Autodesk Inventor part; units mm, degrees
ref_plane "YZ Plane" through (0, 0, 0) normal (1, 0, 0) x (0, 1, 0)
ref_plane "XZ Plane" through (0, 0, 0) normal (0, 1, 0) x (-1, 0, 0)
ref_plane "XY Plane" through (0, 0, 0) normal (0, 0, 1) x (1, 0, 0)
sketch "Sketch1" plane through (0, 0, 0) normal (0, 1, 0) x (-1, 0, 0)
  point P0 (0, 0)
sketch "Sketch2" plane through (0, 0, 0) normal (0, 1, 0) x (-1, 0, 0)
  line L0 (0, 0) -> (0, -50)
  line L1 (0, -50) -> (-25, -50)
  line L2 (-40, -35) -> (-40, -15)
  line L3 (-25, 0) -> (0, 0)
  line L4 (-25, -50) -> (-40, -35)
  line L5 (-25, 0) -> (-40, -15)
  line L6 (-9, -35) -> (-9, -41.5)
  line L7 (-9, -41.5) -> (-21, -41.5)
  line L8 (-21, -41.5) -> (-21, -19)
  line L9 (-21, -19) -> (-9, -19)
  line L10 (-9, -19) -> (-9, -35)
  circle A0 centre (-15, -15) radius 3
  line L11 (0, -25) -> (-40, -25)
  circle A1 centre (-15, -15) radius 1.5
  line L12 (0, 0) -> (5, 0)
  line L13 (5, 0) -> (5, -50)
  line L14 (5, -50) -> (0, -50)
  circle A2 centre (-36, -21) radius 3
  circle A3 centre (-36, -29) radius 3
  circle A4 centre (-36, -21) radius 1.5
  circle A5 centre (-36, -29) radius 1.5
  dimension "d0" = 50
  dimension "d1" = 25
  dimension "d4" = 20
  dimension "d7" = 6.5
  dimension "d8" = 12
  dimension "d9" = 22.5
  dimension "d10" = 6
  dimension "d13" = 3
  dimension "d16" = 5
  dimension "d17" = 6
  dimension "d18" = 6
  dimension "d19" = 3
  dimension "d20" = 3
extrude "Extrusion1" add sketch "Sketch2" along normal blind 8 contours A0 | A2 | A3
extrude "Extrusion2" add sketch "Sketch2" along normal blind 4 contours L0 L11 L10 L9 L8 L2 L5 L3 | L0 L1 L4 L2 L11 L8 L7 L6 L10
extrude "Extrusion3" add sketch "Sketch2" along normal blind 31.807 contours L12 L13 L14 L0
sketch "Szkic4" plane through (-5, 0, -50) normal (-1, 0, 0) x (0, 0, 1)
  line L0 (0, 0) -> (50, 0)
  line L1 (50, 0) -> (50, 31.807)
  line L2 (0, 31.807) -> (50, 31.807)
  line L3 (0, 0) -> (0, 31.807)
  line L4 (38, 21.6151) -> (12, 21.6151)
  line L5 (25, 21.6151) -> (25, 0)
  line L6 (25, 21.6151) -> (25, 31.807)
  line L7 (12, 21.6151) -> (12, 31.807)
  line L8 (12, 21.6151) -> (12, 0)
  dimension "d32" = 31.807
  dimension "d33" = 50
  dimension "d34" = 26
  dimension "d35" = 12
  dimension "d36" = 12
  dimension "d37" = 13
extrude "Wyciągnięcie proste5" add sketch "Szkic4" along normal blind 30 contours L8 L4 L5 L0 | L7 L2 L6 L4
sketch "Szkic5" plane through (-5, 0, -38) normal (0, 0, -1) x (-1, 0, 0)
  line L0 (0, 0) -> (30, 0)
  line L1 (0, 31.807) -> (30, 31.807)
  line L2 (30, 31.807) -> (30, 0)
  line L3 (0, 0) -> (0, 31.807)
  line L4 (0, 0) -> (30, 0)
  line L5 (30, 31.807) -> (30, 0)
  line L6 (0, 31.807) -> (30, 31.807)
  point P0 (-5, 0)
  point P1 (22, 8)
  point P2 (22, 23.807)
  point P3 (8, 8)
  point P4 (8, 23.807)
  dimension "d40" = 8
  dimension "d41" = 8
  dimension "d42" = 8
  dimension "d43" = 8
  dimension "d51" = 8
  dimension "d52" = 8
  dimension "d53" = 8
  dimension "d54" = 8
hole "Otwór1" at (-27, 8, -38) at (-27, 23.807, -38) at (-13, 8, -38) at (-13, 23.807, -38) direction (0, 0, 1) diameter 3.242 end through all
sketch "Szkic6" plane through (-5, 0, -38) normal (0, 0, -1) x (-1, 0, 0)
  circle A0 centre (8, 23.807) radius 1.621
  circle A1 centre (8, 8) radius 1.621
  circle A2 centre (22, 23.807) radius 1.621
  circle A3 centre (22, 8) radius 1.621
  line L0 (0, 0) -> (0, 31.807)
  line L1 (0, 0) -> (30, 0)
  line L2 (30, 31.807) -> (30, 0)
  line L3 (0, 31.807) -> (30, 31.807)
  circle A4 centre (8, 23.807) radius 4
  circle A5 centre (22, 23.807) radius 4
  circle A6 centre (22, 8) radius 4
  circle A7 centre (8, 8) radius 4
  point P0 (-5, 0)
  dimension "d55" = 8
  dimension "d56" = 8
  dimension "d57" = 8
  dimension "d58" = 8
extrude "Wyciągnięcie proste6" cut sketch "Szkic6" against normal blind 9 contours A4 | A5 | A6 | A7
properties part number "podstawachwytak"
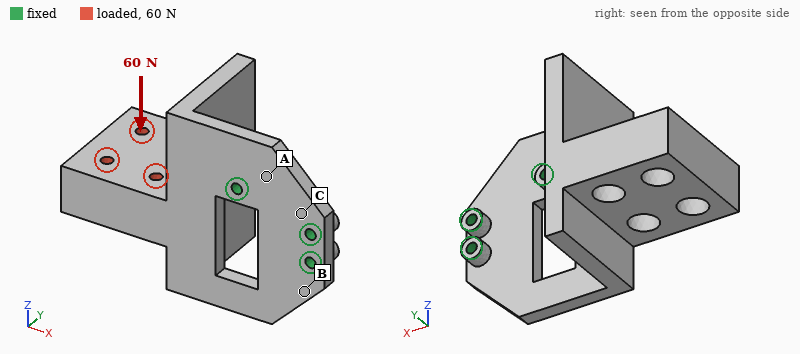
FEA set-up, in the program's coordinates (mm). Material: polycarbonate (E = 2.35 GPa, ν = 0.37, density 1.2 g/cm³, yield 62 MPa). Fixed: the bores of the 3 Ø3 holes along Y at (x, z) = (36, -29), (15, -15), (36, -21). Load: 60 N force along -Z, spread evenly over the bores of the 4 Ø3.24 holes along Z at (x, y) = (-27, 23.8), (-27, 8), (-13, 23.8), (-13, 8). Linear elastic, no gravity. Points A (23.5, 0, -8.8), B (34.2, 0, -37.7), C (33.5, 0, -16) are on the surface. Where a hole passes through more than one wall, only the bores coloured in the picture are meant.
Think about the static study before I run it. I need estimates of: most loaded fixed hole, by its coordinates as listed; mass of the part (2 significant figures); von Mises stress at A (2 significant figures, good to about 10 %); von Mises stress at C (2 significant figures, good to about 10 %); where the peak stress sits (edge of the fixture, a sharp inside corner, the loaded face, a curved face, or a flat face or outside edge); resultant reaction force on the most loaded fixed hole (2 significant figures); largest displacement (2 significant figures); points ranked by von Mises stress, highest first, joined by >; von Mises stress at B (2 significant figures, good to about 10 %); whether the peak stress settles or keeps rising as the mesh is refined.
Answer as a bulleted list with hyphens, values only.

- (15, -15)
- 30 g
- 3.5 MPa
- 1.4 MPa
- edge of the fixture
- 120 N
- 1.0 mm
- B > A > C
- 6.4 MPa
- keeps rising
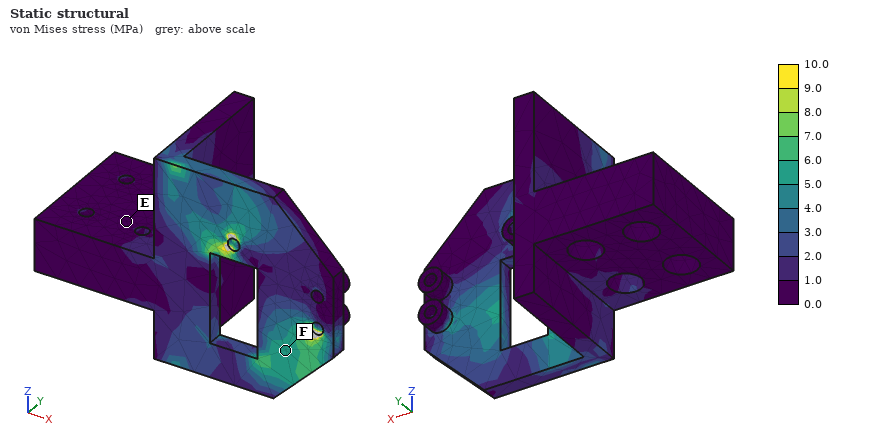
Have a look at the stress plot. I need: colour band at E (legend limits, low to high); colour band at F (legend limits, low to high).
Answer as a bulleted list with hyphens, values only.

- 0.0 to 1.0 MPa
- 5.0 to 6.0 MPa
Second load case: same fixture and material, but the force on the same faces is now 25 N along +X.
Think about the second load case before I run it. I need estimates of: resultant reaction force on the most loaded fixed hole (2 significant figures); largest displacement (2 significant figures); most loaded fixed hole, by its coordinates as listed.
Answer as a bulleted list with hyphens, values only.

- 19 N
- 0.99 mm
- (15, -15)
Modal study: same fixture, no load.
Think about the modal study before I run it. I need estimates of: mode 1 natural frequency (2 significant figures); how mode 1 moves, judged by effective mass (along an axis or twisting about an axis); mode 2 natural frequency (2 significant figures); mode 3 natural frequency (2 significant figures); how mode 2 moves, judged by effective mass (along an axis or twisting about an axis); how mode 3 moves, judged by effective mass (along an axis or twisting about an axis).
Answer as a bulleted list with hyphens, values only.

- 150 Hz
- along Y
- 360 Hz
- 1000 Hz
- along Z
- along Z
